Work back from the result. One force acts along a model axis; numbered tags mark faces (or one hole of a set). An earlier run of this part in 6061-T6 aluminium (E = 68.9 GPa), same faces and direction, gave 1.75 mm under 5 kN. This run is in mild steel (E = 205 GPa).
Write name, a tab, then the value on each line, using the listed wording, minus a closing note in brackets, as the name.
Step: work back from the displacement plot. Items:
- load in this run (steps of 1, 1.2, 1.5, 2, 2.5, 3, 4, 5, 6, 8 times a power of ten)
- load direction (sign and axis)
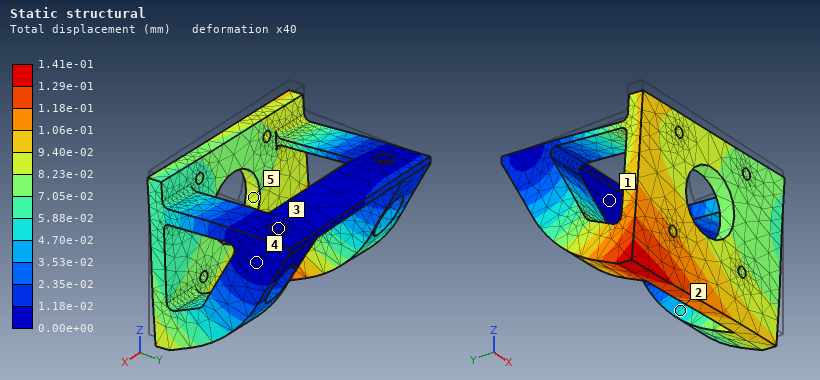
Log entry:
load in this run	1.2 kN
load direction	-Z
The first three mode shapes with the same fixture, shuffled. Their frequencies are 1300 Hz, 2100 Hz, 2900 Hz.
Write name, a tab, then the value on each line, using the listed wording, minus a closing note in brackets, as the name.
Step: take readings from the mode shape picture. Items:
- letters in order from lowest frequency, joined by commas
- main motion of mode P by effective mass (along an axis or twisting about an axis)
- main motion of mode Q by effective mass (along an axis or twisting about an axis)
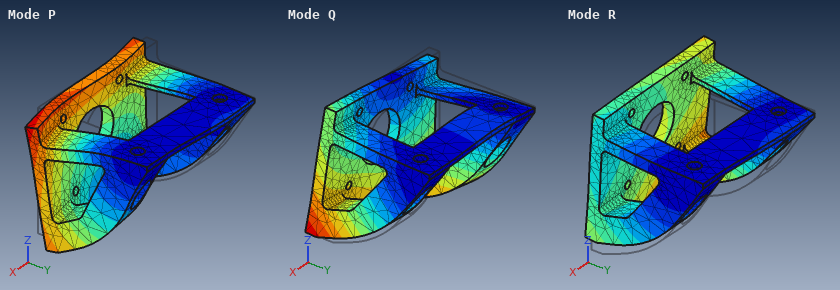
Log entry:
letters in order from lowest frequency, joined by commas	R, Q, P
main motion of mode P by effective mass	along X
main motion of mode Q by effective mass	along X
